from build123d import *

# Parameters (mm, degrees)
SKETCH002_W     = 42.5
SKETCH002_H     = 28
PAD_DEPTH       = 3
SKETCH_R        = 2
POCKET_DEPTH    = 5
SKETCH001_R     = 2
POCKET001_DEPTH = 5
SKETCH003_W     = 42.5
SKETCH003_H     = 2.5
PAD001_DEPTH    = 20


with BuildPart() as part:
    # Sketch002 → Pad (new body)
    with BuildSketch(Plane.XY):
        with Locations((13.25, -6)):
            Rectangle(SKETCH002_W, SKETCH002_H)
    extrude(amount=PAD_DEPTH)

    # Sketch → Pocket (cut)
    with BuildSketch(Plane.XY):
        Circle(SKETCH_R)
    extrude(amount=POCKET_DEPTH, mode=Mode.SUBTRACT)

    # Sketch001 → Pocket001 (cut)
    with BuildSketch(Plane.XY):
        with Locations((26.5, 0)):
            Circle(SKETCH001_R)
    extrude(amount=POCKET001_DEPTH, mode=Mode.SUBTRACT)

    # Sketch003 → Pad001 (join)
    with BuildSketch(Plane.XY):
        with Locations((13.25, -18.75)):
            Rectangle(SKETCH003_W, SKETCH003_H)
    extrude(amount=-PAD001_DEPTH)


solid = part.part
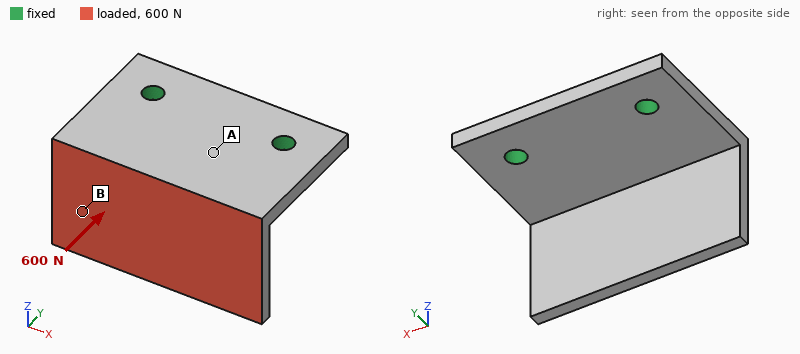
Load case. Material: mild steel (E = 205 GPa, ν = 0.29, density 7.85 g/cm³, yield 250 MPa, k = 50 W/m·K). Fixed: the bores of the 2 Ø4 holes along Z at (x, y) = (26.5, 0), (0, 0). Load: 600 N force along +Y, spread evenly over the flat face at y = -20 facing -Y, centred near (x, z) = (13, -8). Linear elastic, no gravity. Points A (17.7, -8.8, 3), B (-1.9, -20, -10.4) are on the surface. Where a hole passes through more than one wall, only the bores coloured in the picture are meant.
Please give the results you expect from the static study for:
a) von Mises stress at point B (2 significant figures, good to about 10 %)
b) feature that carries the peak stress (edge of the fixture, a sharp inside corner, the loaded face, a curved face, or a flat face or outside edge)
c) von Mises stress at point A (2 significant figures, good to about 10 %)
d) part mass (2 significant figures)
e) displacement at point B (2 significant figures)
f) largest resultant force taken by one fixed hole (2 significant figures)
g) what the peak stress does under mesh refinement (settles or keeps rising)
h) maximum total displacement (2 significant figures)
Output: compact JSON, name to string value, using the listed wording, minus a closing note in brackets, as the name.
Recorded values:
{"von Mises stress at point B": "26 MPa", "feature that carries the peak stress": "edge of the fixture", "von Mises stress at point A": "77 MPa", "part mass": "44 g", "displacement at point B": "0.11 mm", "largest resultant force taken by one fixed hole": "300 N", "what the peak stress does under mesh refinement": "keeps rising", "maximum total displacement": "0.18 mm"}
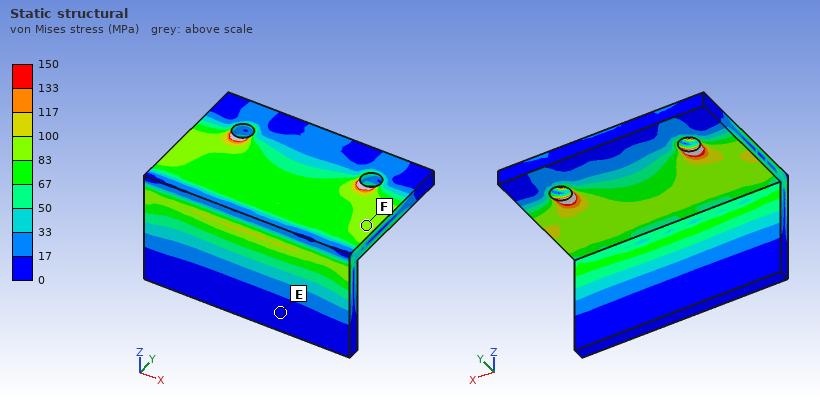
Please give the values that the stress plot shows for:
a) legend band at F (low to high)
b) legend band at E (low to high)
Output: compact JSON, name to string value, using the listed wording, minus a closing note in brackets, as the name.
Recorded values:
{"legend band at F": "83 to 100 MPa", "legend band at E": "0 to 17 MPa"}
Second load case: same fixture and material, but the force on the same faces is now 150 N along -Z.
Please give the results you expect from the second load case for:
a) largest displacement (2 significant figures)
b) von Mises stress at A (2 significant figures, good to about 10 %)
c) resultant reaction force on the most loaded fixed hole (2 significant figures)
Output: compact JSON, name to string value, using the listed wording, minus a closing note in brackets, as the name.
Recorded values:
{"largest displacement": "40 µm", "von Mises stress at A": "22 MPa", "resultant reaction force on the most loaded fixed hole": "75 N"}
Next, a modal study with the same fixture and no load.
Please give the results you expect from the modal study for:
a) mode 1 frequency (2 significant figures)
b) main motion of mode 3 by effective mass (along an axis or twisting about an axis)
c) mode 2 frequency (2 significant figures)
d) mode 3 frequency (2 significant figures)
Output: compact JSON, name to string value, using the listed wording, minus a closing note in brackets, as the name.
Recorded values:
{"mode 1 frequency": "2200 Hz", "main motion of mode 3 by effective mass": "along Z", "mode 2 frequency": "3800 Hz", "mode 3 frequency": "5400 Hz"}
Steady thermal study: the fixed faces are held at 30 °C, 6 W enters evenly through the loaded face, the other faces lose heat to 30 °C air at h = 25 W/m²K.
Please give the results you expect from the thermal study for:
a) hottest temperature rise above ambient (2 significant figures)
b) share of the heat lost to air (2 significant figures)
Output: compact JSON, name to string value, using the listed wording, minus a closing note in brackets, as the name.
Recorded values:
{"hottest temperature rise above ambient": "25 K", "share of the heat lost to air": "17 %"}
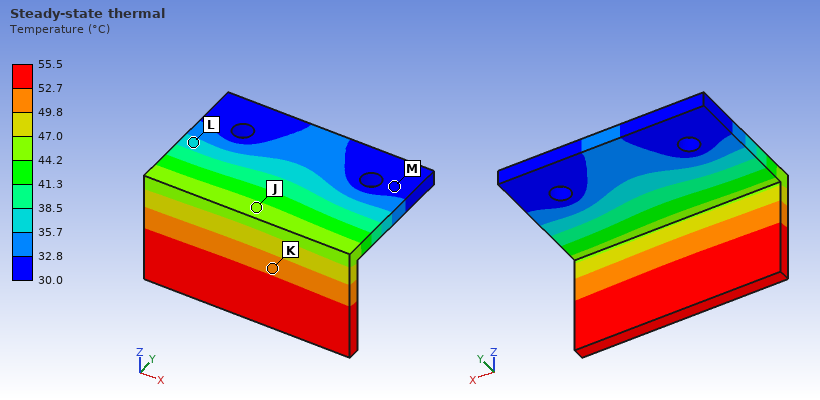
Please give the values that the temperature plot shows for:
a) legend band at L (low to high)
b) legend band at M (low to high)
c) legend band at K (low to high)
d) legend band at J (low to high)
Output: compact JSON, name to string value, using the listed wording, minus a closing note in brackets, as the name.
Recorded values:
{"legend band at L": "35.7 to 38.5 °C", "legend band at M": "30.0 to 32.8 °C", "legend band at K": "49.8 to 52.7 °C", "legend band at J": "44.2 to 47.0 °C"}
